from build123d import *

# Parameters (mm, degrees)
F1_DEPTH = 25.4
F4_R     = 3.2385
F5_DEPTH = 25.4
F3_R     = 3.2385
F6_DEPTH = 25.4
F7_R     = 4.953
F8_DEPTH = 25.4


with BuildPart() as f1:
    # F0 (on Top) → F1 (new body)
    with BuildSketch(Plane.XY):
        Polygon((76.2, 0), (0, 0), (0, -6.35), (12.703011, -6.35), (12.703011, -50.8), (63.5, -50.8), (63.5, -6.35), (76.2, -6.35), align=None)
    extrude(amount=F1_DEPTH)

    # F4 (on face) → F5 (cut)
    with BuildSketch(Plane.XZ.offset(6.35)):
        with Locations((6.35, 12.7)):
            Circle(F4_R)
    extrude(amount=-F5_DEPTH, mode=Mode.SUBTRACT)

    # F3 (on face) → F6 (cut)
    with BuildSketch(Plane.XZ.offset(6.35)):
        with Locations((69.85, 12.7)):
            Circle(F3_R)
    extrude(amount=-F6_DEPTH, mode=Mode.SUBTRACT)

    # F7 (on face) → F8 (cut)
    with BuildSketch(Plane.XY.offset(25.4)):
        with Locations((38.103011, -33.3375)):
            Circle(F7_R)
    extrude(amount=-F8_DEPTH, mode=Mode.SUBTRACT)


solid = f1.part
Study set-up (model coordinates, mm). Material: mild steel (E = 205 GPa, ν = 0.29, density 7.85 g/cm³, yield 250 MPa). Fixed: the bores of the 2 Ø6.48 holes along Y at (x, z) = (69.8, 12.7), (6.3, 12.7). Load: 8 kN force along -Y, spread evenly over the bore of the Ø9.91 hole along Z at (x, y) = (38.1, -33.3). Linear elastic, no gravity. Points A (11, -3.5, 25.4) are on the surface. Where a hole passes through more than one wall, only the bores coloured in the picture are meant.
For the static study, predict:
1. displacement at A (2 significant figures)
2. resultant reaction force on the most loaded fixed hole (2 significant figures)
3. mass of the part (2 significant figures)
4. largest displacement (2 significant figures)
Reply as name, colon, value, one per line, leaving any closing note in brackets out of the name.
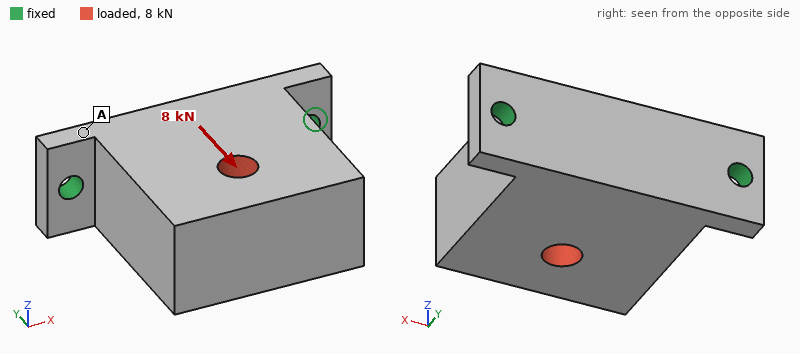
displacement at A: 4.8 µm
resultant reaction force on the most loaded fixed hole: 4.4 kN
mass of the part: 530 g
largest displacement: 8.4 µm
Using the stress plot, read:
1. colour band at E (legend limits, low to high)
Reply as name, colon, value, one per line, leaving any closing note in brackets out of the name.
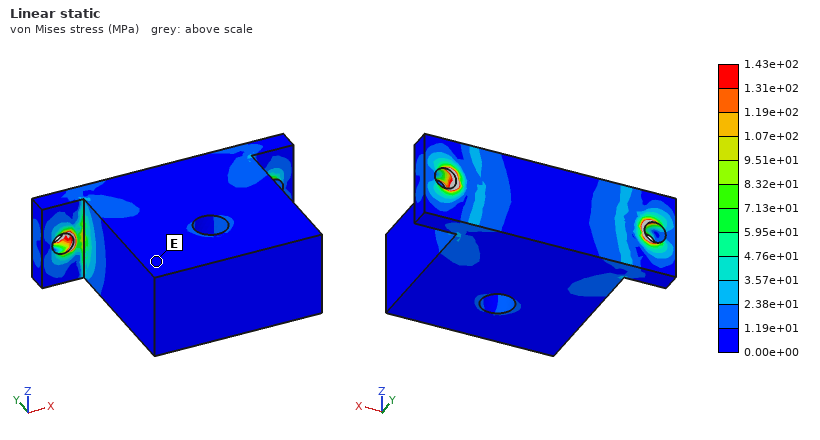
colour band at E: 0.00e+00 to 1.19e+01 MPa
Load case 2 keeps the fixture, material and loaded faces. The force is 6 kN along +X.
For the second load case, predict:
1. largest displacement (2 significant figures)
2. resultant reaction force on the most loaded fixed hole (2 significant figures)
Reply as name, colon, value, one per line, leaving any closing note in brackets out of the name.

largest displacement: 13 µm
resultant reaction force on the most loaded fixed hole: 4.5 kN
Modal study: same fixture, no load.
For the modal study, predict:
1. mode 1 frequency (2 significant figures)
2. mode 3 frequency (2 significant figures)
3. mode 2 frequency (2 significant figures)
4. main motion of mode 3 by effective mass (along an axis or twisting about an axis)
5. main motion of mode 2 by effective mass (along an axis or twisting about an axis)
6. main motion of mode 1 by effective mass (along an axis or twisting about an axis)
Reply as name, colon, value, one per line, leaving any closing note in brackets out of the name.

mode 1 frequency: 1700 Hz
mode 3 frequency: 7500 Hz
mode 2 frequency: 6400 Hz
main motion of mode 3 by effective mass: along Y
main motion of mode 2 by effective mass: along X
main motion of mode 1 by effective mass: along Z
